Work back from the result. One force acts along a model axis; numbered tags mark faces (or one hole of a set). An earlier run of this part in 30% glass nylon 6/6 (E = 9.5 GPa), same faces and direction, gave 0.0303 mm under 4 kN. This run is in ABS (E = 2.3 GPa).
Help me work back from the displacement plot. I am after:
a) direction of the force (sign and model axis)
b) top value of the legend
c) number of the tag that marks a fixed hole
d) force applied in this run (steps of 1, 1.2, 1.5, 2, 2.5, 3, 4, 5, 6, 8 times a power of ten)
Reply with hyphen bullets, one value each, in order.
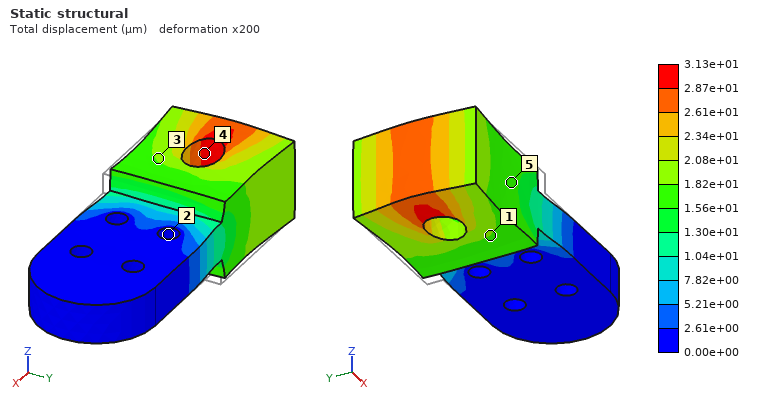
- -X
- 3.13e+01 µm
- 2
- 1 kN
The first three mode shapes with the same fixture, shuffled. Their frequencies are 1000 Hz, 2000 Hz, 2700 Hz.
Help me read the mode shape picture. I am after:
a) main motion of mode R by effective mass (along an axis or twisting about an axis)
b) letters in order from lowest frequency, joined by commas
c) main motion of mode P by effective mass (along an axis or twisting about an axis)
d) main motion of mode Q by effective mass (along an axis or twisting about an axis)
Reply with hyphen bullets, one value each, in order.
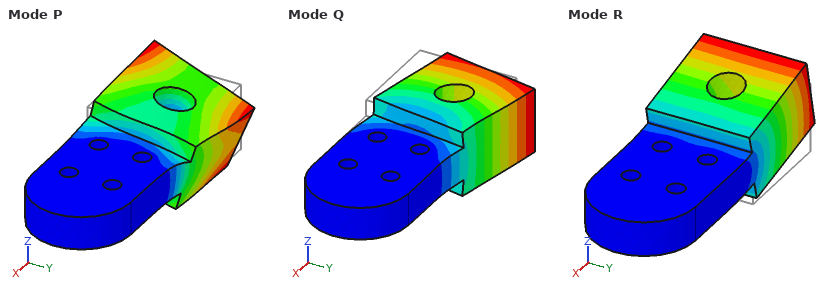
- along Z
- R, Q, P
- twisting about X
- along Y
